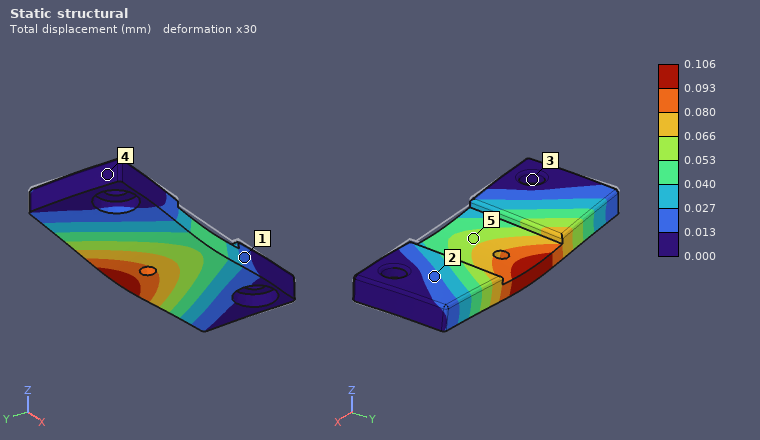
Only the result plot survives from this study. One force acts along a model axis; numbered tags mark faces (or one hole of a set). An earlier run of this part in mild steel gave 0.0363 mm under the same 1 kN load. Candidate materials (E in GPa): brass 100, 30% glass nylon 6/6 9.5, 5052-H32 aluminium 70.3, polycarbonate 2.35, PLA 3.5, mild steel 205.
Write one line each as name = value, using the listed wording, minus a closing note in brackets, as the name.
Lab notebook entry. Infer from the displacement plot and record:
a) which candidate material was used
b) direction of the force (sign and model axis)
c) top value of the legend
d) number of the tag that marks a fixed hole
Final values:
which candidate material was used = 5052-H32 aluminium
direction of the force = -Z
top value of the legend = 0.106 mm
number of the tag that marks a fixed hole = 3
